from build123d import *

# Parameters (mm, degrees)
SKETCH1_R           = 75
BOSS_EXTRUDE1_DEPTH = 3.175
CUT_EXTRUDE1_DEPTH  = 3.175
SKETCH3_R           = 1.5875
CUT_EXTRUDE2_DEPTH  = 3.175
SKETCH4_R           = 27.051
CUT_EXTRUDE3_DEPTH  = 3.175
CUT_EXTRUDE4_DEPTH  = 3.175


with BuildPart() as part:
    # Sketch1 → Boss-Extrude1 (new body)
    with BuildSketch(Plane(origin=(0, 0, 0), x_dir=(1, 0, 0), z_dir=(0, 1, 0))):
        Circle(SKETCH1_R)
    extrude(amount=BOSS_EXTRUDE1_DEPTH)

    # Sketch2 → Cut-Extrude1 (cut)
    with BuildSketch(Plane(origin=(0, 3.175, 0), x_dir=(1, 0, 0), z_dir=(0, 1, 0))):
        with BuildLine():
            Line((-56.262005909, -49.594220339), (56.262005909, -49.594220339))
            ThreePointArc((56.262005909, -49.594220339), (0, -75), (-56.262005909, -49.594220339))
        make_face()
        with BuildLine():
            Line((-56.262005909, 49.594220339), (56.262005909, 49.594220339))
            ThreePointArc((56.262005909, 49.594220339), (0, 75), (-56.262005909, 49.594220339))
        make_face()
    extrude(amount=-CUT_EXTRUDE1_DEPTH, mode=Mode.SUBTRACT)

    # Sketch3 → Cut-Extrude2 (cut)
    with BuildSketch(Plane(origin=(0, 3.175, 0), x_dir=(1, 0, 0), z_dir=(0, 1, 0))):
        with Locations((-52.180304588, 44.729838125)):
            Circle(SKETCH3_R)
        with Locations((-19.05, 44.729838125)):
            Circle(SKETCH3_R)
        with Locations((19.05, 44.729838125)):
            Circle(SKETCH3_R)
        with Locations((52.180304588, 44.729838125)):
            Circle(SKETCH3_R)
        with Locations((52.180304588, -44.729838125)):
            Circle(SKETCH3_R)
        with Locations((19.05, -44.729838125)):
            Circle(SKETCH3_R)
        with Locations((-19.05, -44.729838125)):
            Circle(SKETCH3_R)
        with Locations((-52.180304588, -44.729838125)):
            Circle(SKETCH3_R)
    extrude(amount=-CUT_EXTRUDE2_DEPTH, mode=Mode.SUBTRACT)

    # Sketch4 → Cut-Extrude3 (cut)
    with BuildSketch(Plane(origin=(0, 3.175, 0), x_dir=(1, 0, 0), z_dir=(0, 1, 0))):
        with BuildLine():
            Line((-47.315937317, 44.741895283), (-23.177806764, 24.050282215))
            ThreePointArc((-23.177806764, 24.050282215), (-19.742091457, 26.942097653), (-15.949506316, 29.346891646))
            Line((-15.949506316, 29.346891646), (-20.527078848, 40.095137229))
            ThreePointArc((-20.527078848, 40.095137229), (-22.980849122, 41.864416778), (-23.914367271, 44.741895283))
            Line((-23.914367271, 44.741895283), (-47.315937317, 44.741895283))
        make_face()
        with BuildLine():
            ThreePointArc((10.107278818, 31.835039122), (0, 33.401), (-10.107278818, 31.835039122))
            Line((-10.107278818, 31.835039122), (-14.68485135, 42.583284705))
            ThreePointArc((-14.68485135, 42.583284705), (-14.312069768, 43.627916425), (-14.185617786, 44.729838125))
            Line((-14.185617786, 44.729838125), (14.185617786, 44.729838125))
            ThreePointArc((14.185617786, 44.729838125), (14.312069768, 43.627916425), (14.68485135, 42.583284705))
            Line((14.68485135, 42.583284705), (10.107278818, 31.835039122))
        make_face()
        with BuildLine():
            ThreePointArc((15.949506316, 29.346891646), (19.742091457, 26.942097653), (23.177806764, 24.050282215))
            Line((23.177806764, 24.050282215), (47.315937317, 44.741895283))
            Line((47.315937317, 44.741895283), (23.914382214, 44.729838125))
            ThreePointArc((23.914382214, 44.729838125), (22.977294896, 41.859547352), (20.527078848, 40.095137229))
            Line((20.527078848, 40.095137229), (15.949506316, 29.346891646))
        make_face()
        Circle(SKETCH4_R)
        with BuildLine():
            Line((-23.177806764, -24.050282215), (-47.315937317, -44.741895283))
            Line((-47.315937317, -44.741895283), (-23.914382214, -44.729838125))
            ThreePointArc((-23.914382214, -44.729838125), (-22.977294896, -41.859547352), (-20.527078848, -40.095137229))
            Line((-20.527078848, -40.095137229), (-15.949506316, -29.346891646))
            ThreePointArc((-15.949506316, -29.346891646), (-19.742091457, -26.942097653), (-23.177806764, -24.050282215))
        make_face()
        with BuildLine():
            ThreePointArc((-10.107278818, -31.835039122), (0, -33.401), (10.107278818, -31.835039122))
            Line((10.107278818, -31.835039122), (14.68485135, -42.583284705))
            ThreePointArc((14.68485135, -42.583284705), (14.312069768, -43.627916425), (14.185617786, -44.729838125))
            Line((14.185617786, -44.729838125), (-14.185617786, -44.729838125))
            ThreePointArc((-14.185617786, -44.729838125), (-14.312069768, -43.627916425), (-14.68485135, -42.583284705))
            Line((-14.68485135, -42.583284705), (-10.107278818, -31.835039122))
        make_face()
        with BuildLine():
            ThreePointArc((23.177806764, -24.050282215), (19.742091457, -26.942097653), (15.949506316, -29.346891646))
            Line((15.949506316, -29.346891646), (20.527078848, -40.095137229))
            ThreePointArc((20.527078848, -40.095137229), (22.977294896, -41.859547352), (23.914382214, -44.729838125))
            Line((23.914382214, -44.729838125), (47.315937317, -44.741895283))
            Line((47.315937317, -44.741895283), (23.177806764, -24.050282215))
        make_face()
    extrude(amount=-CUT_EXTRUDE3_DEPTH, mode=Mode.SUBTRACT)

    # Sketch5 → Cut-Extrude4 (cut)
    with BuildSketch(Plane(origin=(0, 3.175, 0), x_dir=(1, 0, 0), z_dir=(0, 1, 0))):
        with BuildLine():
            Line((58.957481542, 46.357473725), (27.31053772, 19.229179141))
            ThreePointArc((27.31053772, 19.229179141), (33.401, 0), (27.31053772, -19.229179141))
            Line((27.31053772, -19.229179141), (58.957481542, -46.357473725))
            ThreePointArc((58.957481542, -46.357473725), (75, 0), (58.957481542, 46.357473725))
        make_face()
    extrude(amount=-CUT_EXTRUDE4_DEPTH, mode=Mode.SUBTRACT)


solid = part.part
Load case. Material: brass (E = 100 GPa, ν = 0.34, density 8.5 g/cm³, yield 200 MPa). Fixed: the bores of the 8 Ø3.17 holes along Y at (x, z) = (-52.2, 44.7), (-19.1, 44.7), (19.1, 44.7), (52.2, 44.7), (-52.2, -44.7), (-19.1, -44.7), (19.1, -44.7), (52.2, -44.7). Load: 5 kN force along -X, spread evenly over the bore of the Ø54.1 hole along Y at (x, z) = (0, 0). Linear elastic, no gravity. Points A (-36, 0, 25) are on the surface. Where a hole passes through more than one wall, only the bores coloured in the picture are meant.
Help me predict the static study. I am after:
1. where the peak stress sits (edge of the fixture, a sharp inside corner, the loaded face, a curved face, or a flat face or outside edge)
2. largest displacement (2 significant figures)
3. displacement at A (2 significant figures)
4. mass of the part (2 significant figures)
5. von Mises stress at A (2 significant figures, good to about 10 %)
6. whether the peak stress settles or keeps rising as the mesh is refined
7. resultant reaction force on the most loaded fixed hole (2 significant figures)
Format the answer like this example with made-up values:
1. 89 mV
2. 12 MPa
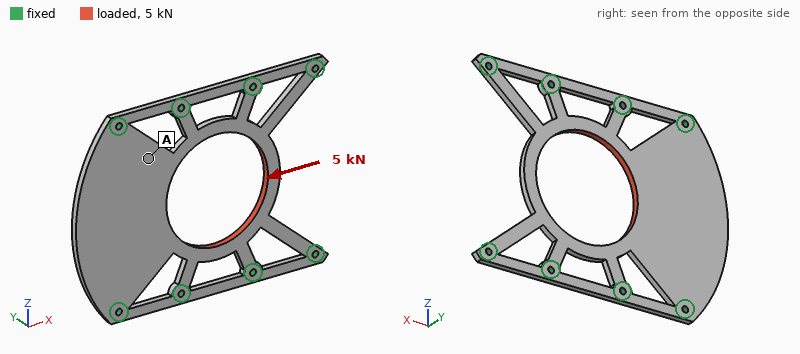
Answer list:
1. edge of the fixture
2. 72 µm
3. 15 µm
4. 180 g
5. 20 MPa
6. keeps rising
7. 1.2 kN
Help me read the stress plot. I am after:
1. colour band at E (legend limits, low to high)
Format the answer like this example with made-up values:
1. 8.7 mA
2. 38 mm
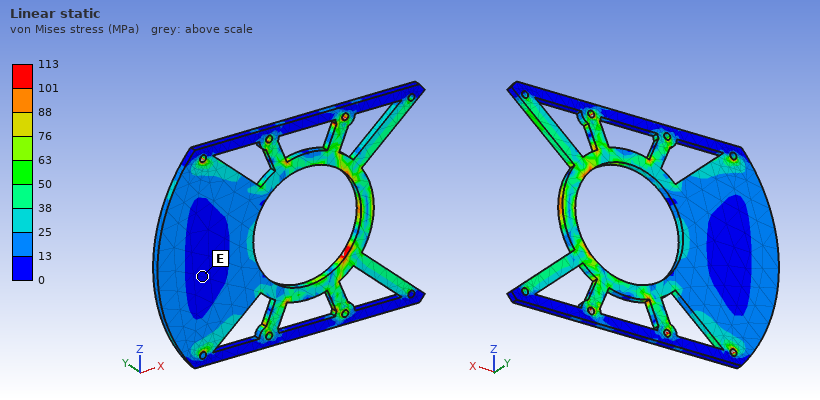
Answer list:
1. 0 to 13 MPa
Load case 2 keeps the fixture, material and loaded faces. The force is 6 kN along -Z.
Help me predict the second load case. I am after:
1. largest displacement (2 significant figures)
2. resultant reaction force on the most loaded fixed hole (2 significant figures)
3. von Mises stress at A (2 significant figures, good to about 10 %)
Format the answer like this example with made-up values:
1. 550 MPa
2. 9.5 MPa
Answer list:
1. 31 µm
2. 1.2 kN
3. 11 MPa
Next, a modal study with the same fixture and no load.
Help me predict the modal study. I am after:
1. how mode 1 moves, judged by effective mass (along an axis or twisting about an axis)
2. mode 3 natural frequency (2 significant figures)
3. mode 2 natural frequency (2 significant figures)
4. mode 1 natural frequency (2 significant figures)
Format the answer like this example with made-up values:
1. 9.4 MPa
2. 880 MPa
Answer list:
1. along Y
2. 1700 Hz
3. 1500 Hz
4. 1100 Hz
